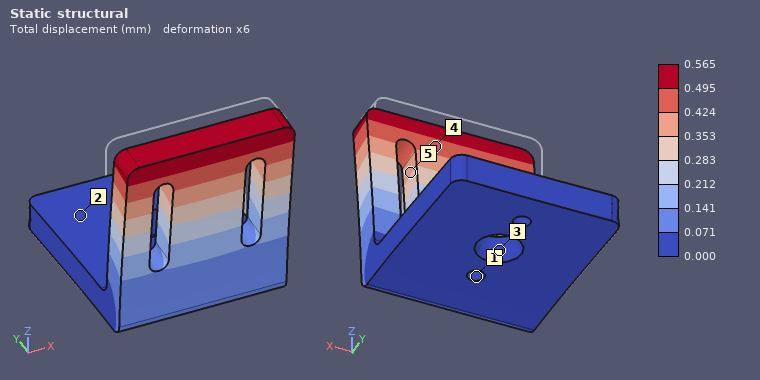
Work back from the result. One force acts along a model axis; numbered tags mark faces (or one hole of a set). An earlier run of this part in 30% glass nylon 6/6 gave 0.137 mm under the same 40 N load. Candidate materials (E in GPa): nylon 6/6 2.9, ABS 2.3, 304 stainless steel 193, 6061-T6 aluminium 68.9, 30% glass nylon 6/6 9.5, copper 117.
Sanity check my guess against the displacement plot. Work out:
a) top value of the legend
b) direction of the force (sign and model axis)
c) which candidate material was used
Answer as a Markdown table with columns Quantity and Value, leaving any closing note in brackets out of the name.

| Quantity | Value |
|---|---|
| top value of the legend | 0.565 mm |
| direction of the force | -Y |
| which candidate material was used | ABS |
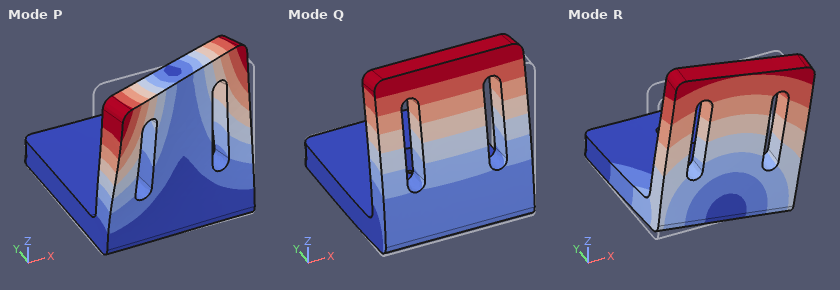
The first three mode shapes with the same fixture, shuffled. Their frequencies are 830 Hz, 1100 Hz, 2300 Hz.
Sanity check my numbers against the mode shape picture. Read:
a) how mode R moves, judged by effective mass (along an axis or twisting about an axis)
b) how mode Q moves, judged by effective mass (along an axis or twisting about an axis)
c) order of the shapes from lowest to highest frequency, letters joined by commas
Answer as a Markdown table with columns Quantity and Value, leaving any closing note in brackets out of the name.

| Quantity | Value |
|---|---|
| how mode R moves, judged by effective mass | along X |
| how mode Q moves, judged by effective mass | along Y |
| order of the shapes from lowest to highest frequency, letters joined by commas | Q, R, P |
